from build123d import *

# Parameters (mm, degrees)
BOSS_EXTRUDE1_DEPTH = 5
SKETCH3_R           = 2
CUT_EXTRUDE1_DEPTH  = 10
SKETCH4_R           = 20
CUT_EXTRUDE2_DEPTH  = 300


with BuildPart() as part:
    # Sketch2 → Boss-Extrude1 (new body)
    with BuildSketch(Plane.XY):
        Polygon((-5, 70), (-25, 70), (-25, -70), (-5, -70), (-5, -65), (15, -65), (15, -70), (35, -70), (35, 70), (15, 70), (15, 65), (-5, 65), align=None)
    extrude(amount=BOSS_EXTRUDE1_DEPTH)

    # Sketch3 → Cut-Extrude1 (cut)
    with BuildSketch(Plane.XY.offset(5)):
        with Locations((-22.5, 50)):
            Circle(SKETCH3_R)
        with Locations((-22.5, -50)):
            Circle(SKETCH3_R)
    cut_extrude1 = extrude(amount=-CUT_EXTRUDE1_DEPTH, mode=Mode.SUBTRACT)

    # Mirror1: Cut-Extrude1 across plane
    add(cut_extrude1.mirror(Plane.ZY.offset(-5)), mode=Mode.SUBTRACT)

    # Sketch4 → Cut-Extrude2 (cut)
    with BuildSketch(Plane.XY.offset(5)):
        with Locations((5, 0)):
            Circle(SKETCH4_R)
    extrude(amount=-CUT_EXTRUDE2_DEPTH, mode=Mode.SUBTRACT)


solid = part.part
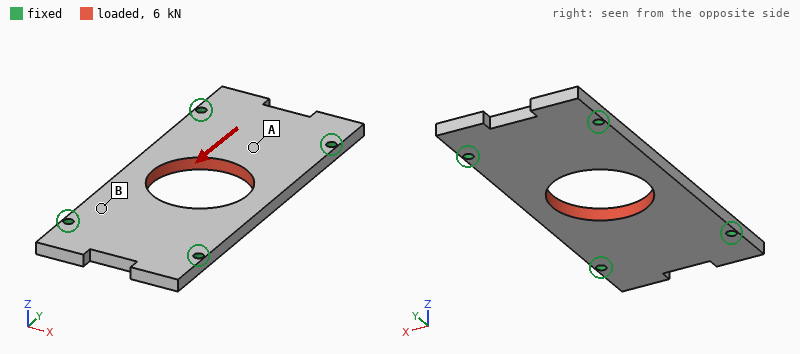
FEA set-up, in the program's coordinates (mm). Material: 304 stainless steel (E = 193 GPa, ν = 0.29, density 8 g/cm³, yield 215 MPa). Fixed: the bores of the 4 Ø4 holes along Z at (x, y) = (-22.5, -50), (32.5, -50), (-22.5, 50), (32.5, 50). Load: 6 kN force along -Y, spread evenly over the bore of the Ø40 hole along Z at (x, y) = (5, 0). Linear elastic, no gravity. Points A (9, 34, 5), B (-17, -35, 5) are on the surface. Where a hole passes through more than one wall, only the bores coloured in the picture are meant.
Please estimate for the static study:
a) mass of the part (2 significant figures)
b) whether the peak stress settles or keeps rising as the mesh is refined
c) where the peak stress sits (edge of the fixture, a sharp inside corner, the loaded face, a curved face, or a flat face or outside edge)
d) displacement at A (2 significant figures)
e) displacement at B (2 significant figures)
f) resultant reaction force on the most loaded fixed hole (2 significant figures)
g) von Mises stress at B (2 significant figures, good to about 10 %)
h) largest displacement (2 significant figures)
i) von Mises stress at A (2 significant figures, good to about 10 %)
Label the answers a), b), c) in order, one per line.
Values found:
a) 280 g
b) keeps rising
c) edge of the fixture
d) 2.6 µm
e) 1.8 µm
f) 1.5 kN
g) 15 MPa
h) 3.7 µm
i) 6.0 MPa
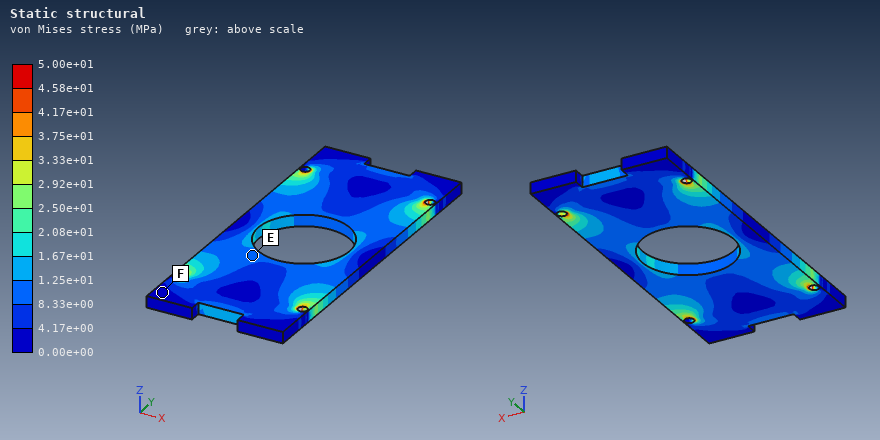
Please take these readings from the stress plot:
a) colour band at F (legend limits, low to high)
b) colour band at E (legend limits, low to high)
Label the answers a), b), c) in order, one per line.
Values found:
a) 0.00e+00 to 4.17e+00 MPa
b) 8.33e+00 to 1.25e+01 MPa
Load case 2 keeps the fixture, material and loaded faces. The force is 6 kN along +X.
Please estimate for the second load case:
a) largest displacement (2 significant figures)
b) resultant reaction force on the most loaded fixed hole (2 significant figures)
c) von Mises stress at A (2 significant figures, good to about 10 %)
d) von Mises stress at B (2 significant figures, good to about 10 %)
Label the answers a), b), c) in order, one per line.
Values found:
a) 11 µm
b) 1.9 kN
c) 26 MPa
d) 15 MPa
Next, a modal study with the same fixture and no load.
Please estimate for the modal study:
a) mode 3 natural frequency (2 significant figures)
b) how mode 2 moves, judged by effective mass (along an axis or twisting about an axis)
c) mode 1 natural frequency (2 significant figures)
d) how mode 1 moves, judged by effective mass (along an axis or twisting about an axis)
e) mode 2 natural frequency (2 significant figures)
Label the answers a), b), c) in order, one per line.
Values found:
a) 4800 Hz
b) twisting about Y
c) 2300 Hz
d) along Z
e) 3600 Hz
